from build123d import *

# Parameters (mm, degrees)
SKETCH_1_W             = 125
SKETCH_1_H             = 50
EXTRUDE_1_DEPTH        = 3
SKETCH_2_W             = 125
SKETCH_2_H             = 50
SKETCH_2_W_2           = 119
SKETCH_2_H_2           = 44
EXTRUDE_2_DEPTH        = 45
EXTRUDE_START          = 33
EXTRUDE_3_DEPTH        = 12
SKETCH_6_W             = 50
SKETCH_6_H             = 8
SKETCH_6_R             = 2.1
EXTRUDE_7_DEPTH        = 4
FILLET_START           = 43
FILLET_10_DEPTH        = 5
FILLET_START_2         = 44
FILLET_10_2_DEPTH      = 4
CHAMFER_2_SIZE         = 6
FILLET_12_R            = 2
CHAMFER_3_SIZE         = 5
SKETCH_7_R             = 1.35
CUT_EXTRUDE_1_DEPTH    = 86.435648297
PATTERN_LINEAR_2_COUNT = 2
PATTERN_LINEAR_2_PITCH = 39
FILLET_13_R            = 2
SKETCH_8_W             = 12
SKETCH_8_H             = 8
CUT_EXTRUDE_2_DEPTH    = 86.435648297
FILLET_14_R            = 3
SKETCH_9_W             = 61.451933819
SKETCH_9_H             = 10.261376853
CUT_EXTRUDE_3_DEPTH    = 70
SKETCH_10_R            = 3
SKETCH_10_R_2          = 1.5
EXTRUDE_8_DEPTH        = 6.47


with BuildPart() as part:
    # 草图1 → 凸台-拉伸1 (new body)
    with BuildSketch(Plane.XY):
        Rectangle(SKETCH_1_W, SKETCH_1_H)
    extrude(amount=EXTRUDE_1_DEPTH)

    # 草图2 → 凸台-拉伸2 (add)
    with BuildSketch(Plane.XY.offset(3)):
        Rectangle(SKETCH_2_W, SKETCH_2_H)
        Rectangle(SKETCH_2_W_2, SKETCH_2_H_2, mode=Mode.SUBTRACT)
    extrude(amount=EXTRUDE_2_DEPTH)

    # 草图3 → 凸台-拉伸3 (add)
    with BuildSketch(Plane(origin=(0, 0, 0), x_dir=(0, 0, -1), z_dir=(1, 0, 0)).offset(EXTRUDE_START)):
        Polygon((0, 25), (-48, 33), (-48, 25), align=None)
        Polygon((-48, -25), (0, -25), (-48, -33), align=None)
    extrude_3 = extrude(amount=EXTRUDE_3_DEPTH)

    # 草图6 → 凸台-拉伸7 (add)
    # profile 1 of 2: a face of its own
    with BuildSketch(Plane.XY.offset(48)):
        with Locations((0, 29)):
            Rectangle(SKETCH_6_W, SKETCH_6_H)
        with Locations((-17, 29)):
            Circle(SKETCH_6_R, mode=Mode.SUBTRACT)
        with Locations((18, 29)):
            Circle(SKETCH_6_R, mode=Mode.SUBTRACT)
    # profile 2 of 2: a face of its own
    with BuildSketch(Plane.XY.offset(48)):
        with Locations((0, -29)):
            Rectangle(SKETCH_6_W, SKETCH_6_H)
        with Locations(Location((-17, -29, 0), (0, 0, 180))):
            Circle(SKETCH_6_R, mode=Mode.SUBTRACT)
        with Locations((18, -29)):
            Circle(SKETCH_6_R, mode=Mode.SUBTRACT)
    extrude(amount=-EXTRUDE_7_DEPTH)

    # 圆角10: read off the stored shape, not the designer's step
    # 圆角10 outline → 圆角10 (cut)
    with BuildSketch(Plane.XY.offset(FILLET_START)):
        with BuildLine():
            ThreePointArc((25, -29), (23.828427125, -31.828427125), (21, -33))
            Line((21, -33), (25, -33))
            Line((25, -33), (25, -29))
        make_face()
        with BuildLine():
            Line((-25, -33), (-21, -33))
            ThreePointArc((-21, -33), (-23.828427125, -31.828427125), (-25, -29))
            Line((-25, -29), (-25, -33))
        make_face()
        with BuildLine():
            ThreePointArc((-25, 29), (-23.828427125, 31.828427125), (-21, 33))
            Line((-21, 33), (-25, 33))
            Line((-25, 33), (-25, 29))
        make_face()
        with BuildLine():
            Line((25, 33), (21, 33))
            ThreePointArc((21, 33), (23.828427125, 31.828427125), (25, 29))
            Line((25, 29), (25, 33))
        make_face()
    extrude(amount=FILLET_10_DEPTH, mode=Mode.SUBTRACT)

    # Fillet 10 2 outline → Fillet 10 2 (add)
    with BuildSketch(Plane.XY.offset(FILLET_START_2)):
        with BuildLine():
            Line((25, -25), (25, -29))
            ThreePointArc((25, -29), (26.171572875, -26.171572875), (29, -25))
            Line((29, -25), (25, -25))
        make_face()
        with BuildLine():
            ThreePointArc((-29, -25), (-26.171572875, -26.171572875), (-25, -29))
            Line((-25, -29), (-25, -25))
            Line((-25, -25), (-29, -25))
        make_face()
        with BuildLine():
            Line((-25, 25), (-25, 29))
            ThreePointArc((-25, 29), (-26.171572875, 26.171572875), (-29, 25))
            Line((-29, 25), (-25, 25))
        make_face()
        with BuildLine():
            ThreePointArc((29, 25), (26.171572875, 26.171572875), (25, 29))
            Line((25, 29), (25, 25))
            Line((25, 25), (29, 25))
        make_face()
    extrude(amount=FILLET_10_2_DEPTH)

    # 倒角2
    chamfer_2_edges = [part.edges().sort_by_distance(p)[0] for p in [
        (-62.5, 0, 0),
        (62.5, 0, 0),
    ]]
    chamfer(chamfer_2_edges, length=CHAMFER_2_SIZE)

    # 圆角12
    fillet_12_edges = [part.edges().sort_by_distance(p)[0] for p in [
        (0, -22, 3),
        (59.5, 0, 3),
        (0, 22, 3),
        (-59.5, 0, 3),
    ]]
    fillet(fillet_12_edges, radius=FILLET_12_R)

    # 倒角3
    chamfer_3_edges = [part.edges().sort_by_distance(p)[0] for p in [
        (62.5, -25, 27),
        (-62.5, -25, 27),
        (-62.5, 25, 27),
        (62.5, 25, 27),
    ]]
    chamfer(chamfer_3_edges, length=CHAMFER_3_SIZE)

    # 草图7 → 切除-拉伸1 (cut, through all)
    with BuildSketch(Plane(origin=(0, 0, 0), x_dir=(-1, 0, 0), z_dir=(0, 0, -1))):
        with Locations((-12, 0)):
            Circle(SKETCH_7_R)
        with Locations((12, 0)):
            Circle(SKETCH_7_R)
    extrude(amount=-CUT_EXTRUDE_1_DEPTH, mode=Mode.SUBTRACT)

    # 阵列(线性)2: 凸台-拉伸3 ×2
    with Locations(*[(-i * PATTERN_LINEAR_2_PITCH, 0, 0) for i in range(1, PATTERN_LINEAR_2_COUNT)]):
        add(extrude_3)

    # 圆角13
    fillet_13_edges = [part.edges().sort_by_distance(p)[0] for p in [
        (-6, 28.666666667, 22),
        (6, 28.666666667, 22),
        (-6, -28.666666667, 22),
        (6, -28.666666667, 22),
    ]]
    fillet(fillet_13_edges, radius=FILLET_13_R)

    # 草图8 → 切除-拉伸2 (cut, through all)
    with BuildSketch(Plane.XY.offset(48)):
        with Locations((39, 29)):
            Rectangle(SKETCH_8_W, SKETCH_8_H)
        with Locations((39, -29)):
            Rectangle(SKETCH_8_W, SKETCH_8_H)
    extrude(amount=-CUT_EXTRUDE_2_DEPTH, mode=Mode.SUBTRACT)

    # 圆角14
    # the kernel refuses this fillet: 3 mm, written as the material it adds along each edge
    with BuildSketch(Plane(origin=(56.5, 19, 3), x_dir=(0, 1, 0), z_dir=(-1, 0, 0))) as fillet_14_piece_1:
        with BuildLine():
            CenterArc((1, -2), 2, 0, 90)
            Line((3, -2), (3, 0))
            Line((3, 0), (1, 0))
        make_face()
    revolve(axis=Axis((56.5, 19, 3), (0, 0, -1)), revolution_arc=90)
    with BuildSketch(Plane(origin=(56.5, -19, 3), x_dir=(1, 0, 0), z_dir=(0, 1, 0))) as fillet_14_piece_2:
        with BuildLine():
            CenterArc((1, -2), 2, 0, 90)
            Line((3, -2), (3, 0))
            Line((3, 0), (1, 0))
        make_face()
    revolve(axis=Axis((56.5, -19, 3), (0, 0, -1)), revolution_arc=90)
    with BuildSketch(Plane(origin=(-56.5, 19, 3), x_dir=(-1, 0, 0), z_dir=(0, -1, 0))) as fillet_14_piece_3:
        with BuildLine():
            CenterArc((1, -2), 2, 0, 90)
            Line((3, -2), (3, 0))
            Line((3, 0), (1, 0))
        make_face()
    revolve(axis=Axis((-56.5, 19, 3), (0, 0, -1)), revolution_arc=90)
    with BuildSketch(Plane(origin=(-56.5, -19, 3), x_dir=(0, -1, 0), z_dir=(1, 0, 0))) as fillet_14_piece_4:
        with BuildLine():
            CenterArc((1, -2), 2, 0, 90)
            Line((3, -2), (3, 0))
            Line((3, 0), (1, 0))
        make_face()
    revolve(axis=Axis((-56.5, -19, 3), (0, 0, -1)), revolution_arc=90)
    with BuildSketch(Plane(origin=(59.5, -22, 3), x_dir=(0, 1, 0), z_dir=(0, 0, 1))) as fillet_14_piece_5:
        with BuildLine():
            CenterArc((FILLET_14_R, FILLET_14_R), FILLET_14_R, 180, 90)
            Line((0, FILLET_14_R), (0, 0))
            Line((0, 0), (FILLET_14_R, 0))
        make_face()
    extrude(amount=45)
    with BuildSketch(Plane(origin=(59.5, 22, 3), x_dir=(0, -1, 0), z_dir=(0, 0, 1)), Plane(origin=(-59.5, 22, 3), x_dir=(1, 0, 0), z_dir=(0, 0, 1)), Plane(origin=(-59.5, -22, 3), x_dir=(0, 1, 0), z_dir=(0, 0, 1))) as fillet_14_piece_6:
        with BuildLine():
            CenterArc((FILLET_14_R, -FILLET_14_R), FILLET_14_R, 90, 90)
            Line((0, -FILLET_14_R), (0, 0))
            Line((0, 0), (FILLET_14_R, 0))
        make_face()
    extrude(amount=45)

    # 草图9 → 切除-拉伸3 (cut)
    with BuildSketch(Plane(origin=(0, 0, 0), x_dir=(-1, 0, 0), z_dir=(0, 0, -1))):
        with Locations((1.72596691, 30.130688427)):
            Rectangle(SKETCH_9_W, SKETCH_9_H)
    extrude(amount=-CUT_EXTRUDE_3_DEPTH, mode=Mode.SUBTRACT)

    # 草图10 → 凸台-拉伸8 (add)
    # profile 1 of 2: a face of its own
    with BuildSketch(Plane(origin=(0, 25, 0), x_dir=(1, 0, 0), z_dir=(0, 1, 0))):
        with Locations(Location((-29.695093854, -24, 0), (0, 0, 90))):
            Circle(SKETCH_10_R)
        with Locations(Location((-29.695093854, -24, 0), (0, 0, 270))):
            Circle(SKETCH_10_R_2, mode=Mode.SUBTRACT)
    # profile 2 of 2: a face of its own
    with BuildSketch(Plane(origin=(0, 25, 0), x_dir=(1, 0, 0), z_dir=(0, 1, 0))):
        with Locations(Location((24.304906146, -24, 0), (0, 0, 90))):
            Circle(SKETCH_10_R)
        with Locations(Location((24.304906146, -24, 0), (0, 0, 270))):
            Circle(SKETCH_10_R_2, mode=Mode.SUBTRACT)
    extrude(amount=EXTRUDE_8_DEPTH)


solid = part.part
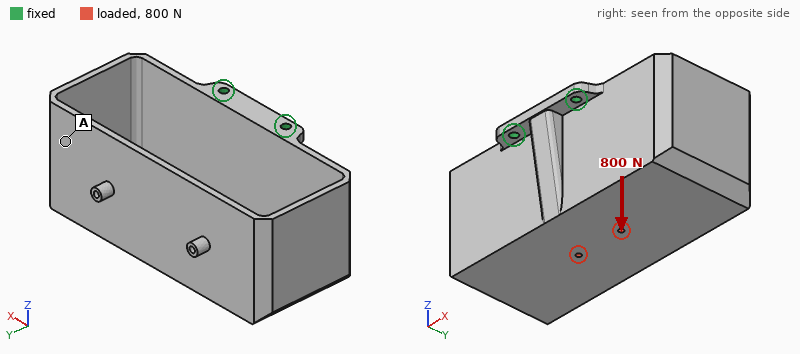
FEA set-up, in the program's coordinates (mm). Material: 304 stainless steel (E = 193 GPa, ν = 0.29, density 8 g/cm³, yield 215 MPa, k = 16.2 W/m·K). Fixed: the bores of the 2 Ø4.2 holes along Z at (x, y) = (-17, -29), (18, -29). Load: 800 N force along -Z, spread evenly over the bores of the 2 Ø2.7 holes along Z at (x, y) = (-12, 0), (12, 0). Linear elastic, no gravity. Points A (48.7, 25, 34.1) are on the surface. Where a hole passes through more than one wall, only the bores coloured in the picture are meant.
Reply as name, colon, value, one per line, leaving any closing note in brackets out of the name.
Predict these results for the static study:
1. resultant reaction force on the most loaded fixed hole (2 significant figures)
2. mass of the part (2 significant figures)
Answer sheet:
resultant reaction force on the most loaded fixed hole: 660 N
mass of the part: 520 g
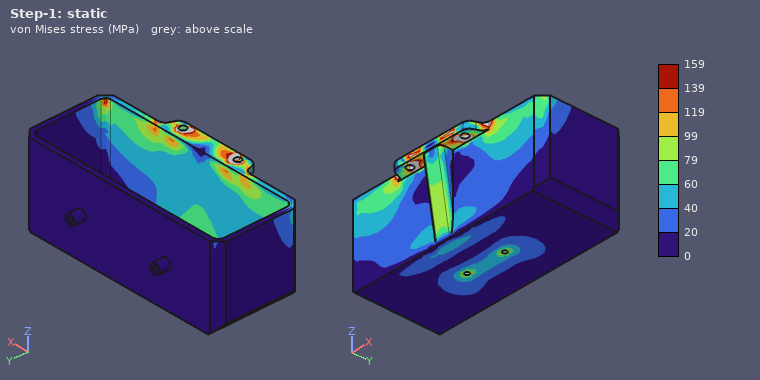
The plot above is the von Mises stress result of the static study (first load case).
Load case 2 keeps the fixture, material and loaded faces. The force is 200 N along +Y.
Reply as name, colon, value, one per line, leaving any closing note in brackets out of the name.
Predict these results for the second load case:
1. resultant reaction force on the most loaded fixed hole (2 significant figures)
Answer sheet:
resultant reaction force on the most loaded fixed hole: 150 N
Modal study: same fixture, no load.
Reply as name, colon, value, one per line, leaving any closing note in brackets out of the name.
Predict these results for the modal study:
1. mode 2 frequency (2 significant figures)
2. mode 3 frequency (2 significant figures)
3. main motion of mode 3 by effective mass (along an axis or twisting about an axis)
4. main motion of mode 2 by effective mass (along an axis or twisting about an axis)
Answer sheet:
mode 2 frequency: 330 Hz
mode 3 frequency: 630 Hz
main motion of mode 3 by effective mass: along Y
main motion of mode 2 by effective mass: along X
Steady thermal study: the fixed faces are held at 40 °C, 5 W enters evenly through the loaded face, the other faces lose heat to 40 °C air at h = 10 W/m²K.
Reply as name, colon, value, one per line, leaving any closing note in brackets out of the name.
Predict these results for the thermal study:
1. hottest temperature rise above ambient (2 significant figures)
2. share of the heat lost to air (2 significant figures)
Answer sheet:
hottest temperature rise above ambient: 40 K
share of the heat lost to air: 83 %
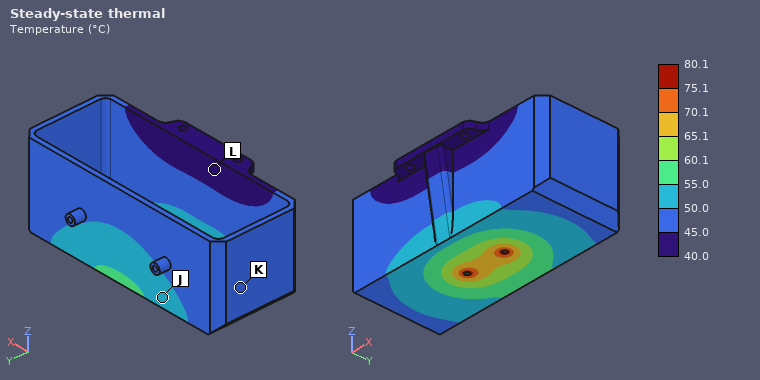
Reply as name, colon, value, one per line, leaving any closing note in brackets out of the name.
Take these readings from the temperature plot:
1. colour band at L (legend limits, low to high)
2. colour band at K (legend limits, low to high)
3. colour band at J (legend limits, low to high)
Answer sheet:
colour band at L: 40.0 to 45.0 °C
colour band at K: 45.0 to 50.0 °C
colour band at J: 50.0 to 55.0 °C
